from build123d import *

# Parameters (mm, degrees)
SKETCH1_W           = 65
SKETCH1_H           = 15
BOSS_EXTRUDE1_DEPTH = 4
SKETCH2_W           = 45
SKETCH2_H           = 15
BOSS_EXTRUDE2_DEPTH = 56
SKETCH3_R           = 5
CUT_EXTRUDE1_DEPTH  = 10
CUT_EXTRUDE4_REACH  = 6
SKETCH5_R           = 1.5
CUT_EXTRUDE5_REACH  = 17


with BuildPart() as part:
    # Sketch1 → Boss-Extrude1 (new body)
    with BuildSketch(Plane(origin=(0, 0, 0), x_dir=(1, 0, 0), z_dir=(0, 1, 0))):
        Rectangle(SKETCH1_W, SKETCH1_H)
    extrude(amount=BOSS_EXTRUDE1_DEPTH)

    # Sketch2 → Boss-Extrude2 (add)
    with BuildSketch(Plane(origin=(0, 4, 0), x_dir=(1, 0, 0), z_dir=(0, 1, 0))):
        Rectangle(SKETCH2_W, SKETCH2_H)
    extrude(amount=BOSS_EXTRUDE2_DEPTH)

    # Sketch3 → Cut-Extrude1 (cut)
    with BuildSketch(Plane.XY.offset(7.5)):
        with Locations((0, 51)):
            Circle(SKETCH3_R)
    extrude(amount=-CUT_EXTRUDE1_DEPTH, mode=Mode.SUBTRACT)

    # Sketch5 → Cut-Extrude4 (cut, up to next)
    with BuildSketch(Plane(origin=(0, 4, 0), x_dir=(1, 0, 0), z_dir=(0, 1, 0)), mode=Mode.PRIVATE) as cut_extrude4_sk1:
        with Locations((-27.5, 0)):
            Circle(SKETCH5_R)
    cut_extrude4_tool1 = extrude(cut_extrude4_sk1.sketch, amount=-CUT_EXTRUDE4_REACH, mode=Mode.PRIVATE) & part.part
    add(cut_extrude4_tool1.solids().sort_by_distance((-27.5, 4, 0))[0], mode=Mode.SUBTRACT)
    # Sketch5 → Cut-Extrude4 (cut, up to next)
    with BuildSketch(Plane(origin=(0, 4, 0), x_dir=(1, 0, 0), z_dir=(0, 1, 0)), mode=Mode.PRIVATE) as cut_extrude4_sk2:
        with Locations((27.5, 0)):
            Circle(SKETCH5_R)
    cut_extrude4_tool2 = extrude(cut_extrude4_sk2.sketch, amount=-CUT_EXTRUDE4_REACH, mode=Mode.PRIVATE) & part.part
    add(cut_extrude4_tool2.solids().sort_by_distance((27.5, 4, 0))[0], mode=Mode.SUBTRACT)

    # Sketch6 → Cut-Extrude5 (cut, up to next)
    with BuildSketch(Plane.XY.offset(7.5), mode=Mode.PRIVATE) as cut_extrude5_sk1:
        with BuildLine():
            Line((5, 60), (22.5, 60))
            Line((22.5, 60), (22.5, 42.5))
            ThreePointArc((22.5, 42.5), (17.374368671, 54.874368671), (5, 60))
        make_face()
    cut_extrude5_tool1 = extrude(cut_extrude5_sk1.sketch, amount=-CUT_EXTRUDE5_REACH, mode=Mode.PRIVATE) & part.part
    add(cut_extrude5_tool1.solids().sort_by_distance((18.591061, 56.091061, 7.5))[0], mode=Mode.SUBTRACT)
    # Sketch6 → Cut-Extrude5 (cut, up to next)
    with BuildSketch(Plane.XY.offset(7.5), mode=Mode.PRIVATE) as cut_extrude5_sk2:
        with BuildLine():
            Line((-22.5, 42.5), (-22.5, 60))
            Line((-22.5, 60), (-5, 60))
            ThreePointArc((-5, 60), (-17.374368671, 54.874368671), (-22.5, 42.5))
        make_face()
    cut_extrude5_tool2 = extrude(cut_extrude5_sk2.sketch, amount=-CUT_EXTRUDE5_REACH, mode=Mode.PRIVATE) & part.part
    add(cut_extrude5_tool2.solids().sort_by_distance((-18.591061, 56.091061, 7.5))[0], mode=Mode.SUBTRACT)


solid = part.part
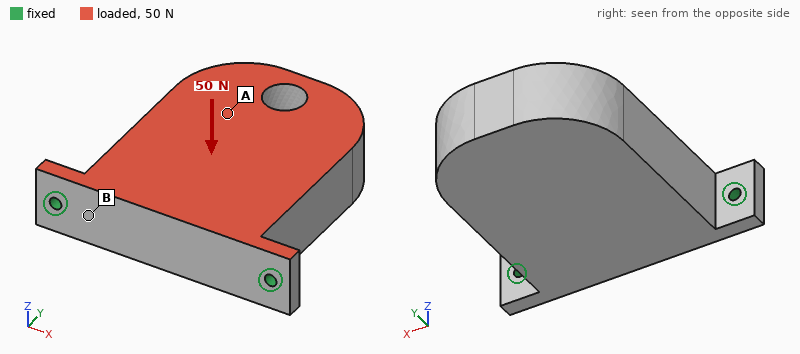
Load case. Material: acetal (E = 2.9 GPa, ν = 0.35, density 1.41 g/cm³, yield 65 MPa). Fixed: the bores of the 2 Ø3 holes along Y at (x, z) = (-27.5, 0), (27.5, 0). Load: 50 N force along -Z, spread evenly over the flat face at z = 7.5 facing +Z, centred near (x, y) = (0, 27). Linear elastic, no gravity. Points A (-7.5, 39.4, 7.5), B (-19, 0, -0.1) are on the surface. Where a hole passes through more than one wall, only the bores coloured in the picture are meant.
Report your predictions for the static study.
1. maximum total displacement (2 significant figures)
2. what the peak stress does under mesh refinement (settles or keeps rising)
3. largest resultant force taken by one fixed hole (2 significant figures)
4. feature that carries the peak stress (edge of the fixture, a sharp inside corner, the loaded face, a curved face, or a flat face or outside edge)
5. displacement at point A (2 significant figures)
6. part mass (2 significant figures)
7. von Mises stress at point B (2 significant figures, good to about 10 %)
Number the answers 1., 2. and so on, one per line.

1. 0.72 mm
2. keeps rising
3. 25 N
4. edge of the fixture
5. 0.47 mm
6. 55 g
7. 2.9 MPa
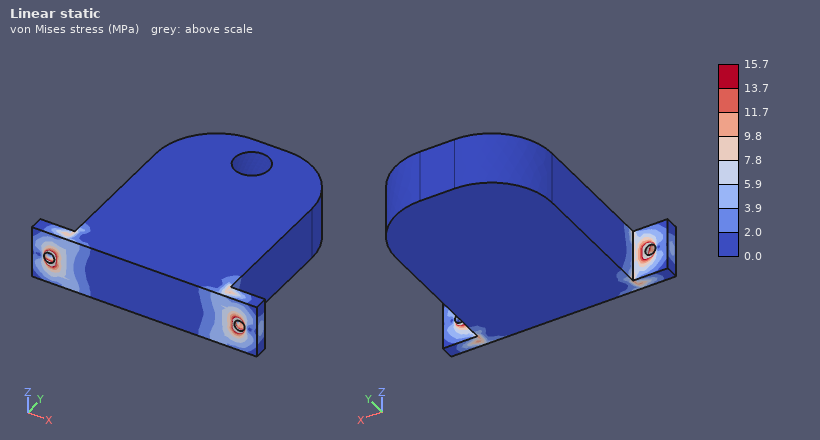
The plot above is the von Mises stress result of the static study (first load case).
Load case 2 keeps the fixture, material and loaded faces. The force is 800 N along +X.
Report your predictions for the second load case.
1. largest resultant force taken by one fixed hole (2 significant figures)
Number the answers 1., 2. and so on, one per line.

1. 580 N
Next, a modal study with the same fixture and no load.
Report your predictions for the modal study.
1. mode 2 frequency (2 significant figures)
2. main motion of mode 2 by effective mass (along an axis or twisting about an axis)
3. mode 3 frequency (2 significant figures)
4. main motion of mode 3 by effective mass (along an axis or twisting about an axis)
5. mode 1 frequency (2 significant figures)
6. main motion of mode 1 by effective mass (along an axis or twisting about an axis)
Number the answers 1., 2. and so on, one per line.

1. 1200 Hz
2. along X
3. 1700 Hz
4. along Y
5. 220 Hz
6. along Z
